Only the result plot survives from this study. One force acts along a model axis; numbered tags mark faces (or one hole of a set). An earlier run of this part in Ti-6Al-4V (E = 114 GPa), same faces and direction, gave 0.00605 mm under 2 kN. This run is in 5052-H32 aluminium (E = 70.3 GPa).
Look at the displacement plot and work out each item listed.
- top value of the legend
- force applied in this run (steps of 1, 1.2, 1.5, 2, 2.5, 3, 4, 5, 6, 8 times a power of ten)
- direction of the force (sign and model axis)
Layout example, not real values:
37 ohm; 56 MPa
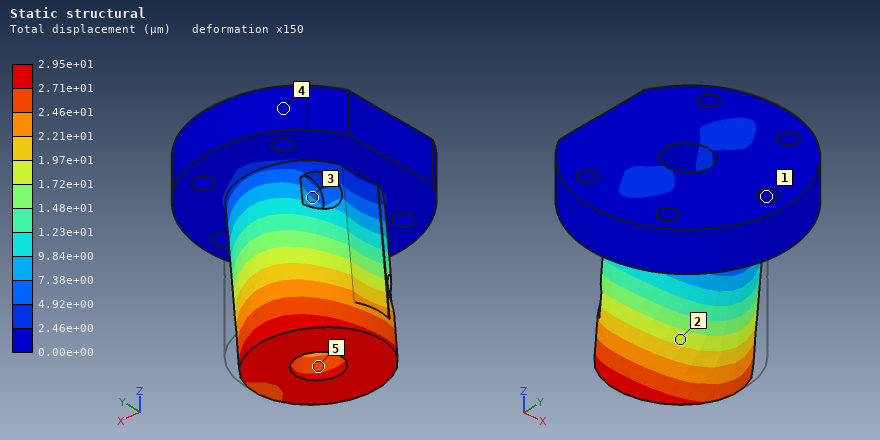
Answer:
2.95e+01 µm; 6 kN; -Y
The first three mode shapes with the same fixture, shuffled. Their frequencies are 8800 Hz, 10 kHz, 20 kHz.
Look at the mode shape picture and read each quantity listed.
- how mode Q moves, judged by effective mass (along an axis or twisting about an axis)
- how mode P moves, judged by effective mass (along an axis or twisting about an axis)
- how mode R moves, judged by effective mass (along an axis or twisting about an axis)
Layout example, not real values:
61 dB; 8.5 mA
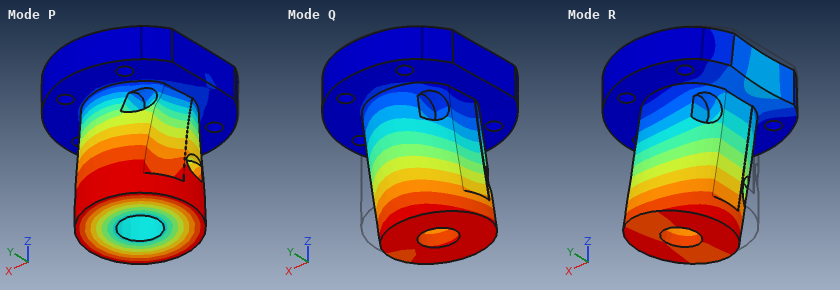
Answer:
along Y; twisting about Z; along X
